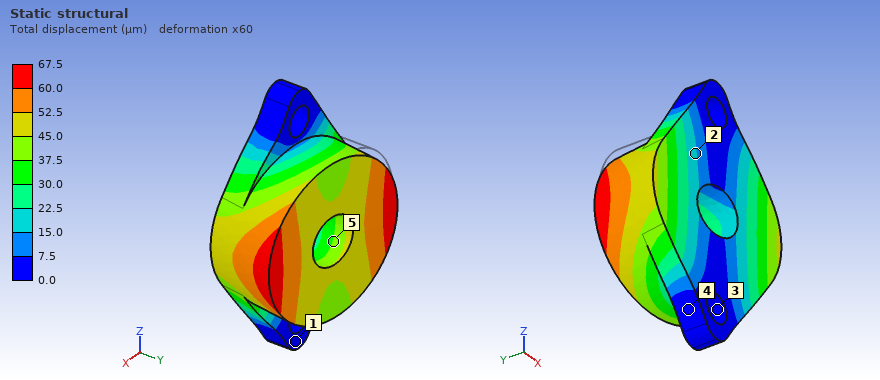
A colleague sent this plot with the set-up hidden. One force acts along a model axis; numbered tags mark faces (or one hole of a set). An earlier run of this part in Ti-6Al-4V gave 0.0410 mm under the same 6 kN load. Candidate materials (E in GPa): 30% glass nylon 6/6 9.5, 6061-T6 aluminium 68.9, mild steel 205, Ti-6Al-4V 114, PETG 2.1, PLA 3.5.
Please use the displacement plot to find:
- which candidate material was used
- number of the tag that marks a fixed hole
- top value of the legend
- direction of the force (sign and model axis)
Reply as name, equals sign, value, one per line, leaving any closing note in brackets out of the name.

which candidate material was used = 6061-T6 aluminium
number of the tag that marks a fixed hole = 3
top value of the legend = 67.5 µm
direction of the force = +X
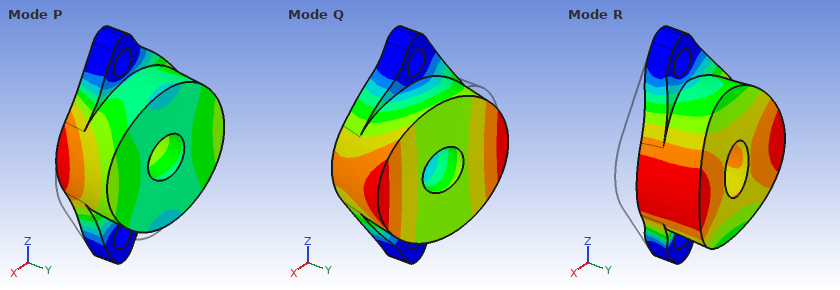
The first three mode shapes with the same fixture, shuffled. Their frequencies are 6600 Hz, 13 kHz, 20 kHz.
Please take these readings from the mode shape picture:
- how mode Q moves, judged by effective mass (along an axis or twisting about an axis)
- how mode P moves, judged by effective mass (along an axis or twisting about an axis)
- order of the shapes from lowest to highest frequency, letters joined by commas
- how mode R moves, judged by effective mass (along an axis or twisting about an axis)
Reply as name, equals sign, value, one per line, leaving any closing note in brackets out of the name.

how mode Q moves, judged by effective mass = along X
how mode P moves, judged by effective mass = along X
order of the shapes from lowest to highest frequency, letters joined by commas = Q, R, P
how mode R moves, judged by effective mass = along Y
